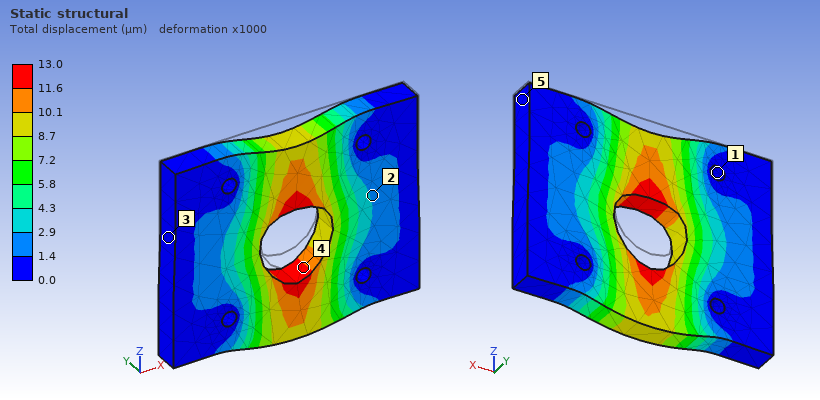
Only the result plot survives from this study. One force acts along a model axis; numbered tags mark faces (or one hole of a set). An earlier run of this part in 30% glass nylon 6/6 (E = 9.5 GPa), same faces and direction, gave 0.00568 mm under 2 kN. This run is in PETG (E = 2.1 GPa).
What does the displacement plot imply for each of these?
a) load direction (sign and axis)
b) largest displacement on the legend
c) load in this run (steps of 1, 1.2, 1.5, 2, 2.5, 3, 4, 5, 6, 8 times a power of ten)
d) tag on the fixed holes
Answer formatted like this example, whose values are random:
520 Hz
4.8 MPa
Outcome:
-Z
13.0 µm
1 kN
1
